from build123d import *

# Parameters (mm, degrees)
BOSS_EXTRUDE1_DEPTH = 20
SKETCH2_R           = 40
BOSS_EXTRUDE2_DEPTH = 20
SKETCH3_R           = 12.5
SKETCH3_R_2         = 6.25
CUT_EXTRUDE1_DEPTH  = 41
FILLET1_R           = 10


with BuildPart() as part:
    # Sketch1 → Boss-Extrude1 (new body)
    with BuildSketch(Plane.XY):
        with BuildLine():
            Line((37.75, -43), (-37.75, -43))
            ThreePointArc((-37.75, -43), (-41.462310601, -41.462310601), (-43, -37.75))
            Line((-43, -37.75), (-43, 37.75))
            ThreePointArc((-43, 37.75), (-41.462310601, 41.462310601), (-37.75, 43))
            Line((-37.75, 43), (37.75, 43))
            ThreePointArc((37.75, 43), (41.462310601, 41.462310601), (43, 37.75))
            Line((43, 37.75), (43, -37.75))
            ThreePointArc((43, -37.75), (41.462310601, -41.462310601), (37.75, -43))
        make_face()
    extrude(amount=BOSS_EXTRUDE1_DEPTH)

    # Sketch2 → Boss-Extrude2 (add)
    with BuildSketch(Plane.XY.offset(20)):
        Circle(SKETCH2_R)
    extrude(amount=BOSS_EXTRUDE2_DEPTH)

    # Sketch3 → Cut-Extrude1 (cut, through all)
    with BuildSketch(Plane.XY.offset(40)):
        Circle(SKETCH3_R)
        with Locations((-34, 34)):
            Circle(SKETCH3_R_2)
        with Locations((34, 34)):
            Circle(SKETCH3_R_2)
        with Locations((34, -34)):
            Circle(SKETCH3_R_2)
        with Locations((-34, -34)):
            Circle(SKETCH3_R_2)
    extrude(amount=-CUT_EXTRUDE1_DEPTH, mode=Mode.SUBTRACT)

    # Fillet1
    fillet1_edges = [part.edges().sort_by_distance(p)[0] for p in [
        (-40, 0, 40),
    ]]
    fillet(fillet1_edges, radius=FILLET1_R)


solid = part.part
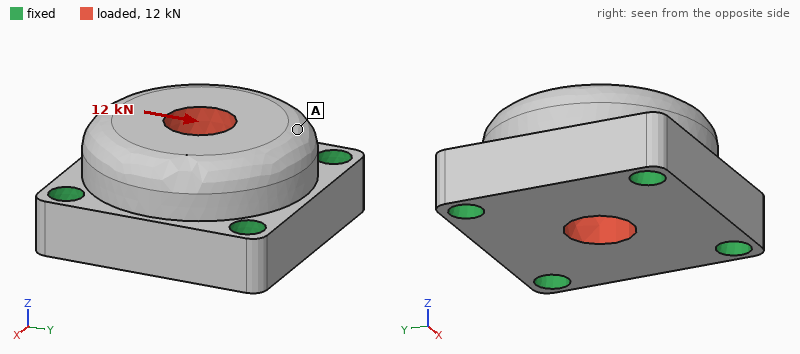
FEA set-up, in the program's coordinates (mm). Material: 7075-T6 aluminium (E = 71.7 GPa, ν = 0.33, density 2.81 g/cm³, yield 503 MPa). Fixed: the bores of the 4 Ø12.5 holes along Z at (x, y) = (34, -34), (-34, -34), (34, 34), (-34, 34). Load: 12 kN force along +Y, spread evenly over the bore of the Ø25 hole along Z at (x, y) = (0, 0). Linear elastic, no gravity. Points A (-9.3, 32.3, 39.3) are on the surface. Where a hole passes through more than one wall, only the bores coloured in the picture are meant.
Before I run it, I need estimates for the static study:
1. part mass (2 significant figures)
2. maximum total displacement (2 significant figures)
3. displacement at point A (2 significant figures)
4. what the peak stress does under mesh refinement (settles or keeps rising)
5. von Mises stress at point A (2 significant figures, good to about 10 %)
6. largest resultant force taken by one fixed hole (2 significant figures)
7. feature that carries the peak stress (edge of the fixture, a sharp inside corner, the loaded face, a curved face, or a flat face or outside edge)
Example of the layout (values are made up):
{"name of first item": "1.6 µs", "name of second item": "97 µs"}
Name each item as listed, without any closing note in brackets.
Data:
{"part mass": "600 g", "maximum total displacement": "4.6 µm", "displacement at point A": "3.7 µm", "what the peak stress does under mesh refinement": "keeps rising", "von Mises stress at point A": "2.5 MPa", "largest resultant force taken by one fixed hole": "3.4 kN", "feature that carries the peak stress": "edge of the fixture"}
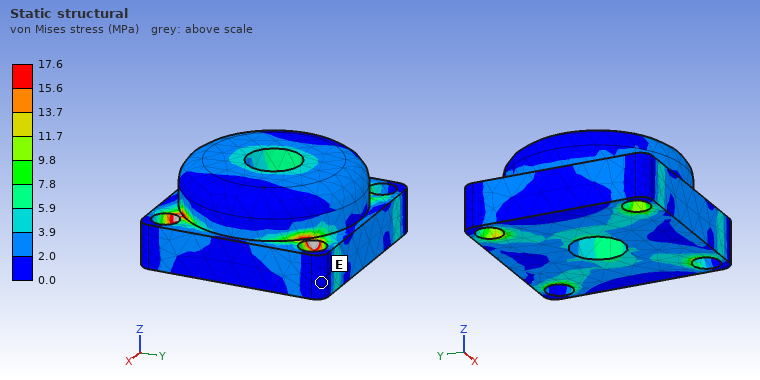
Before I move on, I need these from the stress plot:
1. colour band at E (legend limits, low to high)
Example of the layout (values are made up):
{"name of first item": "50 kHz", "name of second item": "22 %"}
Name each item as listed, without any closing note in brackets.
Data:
{"colour band at E": "0.0 to 2.0 MPa"}
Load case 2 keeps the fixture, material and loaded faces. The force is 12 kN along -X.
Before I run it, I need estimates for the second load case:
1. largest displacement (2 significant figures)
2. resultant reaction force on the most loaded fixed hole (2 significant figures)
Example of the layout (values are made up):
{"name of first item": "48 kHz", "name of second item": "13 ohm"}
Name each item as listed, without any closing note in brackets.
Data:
{"largest displacement": "4.6 µm", "resultant reaction force on the most loaded fixed hole": "3.4 kN"}
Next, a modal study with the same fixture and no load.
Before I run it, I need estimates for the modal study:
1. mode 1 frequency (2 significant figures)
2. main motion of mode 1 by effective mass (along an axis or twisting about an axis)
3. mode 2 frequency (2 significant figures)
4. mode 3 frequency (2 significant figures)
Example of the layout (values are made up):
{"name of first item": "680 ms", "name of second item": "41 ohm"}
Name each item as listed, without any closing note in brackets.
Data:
{"mode 1 frequency": "13 kHz", "main motion of mode 1 by effective mass": "along Z", "mode 2 frequency": "15 kHz", "mode 3 frequency": "15 kHz"}
